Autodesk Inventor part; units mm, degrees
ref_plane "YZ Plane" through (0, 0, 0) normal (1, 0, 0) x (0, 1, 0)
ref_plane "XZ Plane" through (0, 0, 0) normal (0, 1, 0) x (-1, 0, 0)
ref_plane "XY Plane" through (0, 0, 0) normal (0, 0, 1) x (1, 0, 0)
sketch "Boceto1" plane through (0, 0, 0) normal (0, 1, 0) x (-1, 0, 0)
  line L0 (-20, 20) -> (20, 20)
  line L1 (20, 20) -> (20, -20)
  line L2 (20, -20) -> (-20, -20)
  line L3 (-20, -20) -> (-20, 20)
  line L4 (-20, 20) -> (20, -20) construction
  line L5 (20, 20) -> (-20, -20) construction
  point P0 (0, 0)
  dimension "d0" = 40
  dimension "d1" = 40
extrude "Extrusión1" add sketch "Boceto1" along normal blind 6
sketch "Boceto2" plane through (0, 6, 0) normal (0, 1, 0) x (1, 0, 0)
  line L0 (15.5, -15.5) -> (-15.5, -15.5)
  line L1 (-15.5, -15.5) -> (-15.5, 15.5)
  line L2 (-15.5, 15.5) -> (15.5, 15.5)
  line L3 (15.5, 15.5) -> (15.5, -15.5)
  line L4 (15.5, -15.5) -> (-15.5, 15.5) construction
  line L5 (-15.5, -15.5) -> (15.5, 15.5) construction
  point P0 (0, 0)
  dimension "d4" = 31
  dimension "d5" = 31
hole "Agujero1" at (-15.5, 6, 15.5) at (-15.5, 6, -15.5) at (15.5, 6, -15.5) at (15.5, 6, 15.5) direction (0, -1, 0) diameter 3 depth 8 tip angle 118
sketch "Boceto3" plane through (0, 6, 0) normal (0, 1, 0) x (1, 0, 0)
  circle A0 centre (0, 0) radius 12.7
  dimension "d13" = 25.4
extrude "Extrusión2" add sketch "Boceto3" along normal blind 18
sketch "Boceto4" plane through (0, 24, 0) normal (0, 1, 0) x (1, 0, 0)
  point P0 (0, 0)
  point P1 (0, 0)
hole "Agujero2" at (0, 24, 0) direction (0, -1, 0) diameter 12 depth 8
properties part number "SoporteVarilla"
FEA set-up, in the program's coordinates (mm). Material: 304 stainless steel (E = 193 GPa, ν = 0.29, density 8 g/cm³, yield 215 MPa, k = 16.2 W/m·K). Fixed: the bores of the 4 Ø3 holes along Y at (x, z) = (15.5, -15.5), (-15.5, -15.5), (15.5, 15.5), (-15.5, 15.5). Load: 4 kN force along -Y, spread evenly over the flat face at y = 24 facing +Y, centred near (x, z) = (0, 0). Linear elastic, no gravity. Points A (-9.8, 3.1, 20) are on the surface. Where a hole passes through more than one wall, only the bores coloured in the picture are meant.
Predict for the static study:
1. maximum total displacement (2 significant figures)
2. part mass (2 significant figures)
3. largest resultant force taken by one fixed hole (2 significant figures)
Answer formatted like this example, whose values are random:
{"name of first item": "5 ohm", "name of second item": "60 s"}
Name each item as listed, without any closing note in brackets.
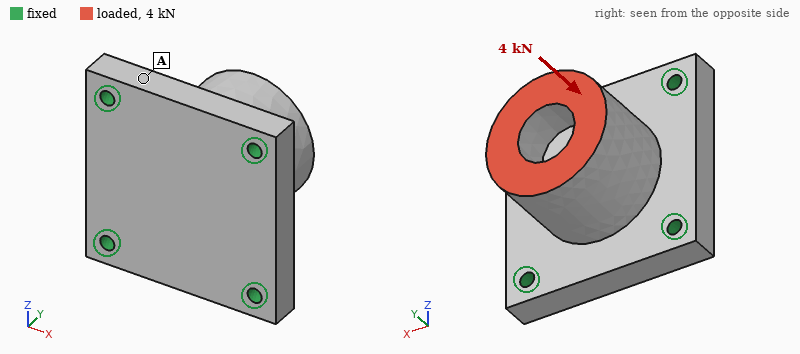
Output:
{"maximum total displacement": "5.9 µm", "part mass": "140 g", "largest resultant force taken by one fixed hole": "1.0 kN"}
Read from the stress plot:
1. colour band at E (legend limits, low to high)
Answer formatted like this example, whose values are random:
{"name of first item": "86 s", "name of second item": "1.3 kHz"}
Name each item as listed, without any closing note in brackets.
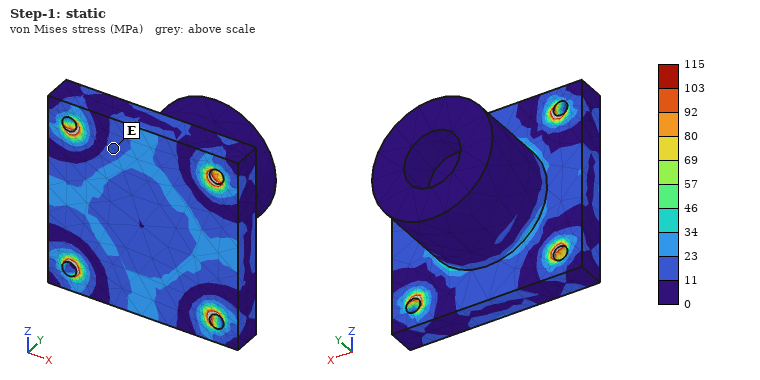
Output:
{"colour band at E": "11 to 23 MPa"}
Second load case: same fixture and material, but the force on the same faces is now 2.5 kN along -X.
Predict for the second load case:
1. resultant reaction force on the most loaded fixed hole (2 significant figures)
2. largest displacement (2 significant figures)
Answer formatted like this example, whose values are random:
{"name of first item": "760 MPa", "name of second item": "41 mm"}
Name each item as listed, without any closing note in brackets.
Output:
{"resultant reaction force on the most loaded fixed hole": "1.2 kN", "largest displacement": "14 µm"}
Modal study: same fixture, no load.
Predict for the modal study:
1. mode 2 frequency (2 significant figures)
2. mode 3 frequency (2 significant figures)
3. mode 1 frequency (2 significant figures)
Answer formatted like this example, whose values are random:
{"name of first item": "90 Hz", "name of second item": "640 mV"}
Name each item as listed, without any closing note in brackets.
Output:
{"mode 2 frequency": "13 kHz", "mode 3 frequency": "14 kHz", "mode 1 frequency": "13 kHz"}
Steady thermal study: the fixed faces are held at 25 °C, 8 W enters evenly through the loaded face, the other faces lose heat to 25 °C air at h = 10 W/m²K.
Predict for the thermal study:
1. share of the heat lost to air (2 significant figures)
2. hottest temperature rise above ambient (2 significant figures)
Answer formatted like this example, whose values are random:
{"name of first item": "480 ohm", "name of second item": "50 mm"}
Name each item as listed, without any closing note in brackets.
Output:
{"share of the heat lost to air": "9.5 %", "hottest temperature rise above ambient": "36 K"}
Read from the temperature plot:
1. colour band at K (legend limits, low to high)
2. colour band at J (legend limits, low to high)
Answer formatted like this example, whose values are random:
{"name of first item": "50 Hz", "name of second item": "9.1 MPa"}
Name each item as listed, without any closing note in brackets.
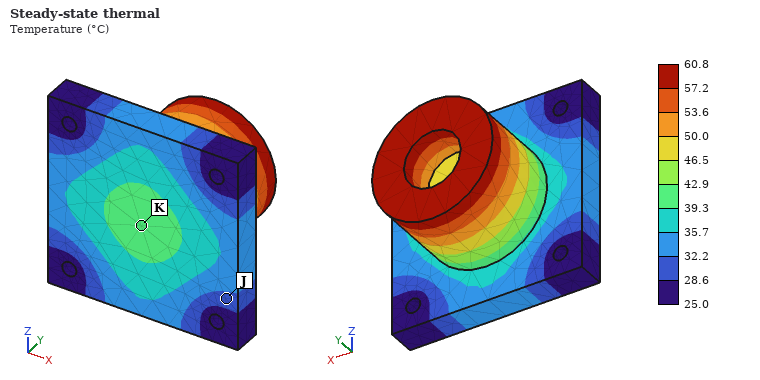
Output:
{"colour band at K": "39.3 to 42.9 °C", "colour band at J": "28.6 to 32.2 °C"}
